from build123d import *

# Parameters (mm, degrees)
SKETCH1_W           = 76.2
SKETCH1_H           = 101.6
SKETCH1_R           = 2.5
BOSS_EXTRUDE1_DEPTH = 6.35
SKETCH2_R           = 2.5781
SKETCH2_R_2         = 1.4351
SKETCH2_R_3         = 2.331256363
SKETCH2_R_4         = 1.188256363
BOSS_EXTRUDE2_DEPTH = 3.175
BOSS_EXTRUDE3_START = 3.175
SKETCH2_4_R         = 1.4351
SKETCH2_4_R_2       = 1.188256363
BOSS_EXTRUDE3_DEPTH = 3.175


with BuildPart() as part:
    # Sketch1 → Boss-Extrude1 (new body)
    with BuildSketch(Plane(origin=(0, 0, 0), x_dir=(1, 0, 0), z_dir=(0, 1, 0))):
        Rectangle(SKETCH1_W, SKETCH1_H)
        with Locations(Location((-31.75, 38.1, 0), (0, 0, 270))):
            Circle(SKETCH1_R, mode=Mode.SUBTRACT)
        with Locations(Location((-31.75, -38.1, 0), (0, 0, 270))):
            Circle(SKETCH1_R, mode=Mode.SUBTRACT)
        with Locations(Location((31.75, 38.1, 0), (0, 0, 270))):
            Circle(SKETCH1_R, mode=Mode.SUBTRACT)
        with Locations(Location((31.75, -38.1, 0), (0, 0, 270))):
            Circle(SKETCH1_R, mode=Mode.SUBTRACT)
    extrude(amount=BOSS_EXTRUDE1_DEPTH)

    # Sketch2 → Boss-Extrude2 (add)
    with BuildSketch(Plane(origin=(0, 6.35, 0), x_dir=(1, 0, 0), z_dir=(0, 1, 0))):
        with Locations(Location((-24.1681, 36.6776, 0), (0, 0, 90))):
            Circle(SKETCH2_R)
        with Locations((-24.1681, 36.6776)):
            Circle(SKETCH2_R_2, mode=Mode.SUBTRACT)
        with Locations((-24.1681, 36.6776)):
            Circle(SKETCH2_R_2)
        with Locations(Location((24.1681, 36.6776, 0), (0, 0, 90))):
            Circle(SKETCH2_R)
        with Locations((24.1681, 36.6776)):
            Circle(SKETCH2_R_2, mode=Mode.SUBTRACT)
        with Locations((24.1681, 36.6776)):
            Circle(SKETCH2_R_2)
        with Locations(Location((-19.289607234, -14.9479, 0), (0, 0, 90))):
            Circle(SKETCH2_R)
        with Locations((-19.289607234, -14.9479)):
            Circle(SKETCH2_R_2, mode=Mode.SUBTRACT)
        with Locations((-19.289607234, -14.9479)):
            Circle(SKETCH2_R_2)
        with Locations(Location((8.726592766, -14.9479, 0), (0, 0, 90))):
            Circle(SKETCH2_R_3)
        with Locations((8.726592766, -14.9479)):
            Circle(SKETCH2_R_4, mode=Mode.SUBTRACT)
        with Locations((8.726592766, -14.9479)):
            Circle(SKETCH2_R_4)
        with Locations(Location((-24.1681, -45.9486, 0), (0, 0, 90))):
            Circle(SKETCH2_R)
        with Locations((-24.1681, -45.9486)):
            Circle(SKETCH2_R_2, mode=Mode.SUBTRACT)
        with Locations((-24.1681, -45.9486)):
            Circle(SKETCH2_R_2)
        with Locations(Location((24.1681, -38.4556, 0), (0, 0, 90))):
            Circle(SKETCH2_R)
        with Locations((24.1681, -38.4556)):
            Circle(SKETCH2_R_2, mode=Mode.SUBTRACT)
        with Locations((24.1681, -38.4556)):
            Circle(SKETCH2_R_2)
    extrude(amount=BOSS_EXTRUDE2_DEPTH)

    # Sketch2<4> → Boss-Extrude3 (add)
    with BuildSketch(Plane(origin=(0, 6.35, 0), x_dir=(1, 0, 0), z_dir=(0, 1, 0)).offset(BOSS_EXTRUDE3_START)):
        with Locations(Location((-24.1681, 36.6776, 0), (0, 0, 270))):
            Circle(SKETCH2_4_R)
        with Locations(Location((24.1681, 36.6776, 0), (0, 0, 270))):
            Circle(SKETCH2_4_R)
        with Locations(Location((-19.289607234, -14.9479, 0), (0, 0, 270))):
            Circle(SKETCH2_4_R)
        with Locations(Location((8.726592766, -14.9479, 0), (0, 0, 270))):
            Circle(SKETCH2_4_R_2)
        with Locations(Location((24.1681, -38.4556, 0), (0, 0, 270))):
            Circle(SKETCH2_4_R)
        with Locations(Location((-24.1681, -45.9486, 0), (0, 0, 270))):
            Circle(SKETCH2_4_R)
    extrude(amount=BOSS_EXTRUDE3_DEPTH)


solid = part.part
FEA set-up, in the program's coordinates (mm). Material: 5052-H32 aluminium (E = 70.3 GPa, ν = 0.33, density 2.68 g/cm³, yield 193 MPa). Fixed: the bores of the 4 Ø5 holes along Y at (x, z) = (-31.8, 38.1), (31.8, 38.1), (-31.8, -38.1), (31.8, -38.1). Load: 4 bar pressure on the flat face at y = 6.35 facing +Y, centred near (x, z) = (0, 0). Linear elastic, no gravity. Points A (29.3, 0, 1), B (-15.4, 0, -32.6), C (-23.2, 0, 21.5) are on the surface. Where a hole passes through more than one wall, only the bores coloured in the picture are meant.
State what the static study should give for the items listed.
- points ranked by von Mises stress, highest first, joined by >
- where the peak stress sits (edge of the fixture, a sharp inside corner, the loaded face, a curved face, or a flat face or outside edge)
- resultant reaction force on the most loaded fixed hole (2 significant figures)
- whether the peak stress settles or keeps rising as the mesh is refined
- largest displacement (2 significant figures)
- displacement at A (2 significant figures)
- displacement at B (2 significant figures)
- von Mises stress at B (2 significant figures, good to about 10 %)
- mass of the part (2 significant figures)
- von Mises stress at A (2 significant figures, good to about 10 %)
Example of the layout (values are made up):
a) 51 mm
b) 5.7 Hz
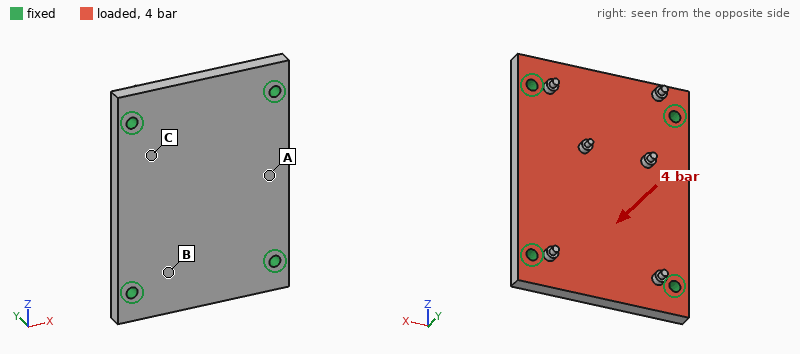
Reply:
a) A > B > C
b) edge of the fixture
c) 760 N
d) keeps rising
e) 45 µm
f) 34 µm
g) 17 µm
h) 9.0 MPa
i) 130 g
j) 17 MPa
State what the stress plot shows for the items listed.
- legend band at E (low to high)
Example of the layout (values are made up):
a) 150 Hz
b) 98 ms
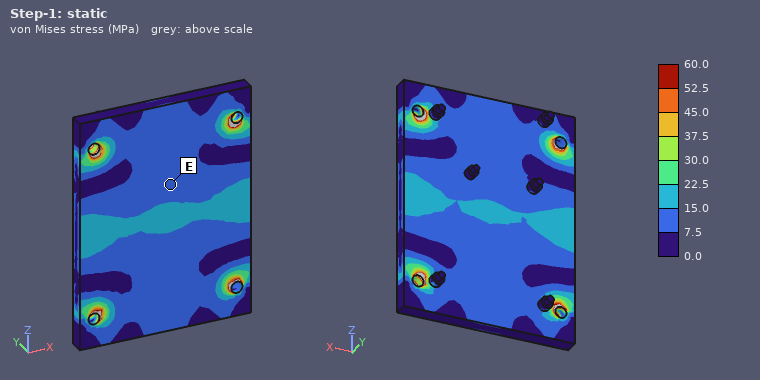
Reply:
a) 7.5 to 15.0 MPa
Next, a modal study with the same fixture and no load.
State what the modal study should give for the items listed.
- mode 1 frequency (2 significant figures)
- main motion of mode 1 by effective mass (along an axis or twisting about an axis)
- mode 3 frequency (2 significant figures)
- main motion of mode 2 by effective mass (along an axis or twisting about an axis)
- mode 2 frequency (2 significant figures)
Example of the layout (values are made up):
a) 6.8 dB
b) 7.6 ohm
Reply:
a) 4300 Hz
b) along Y
c) 7700 Hz
d) twisting about Z
e) 6600 Hz
